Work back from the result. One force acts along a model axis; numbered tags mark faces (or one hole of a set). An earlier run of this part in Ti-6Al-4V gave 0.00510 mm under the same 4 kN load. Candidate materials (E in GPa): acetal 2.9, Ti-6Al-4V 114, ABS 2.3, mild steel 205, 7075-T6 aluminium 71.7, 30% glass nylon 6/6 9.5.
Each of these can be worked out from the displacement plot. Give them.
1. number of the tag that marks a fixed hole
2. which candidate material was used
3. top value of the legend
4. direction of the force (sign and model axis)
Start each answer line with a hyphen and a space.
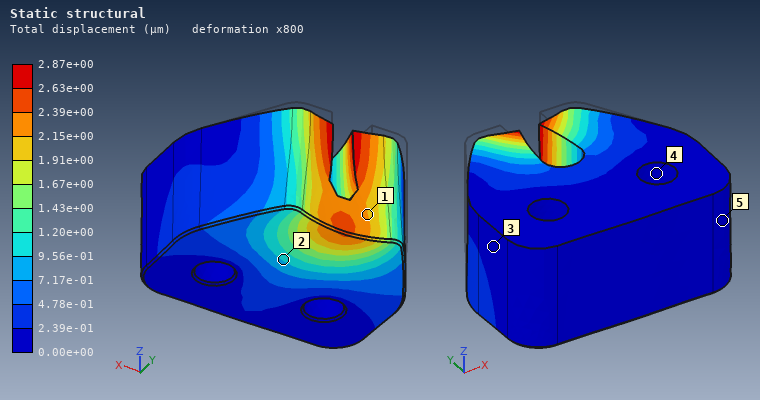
- 4
- mild steel
- 2.87e+00 µm
- -Y
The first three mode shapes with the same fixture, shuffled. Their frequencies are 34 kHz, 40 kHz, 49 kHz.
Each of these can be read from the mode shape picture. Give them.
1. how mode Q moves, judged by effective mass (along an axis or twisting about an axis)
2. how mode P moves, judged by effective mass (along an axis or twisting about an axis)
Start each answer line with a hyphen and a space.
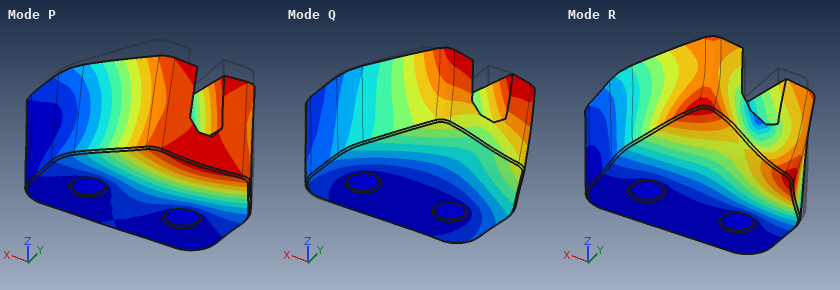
- along X
- along Z
